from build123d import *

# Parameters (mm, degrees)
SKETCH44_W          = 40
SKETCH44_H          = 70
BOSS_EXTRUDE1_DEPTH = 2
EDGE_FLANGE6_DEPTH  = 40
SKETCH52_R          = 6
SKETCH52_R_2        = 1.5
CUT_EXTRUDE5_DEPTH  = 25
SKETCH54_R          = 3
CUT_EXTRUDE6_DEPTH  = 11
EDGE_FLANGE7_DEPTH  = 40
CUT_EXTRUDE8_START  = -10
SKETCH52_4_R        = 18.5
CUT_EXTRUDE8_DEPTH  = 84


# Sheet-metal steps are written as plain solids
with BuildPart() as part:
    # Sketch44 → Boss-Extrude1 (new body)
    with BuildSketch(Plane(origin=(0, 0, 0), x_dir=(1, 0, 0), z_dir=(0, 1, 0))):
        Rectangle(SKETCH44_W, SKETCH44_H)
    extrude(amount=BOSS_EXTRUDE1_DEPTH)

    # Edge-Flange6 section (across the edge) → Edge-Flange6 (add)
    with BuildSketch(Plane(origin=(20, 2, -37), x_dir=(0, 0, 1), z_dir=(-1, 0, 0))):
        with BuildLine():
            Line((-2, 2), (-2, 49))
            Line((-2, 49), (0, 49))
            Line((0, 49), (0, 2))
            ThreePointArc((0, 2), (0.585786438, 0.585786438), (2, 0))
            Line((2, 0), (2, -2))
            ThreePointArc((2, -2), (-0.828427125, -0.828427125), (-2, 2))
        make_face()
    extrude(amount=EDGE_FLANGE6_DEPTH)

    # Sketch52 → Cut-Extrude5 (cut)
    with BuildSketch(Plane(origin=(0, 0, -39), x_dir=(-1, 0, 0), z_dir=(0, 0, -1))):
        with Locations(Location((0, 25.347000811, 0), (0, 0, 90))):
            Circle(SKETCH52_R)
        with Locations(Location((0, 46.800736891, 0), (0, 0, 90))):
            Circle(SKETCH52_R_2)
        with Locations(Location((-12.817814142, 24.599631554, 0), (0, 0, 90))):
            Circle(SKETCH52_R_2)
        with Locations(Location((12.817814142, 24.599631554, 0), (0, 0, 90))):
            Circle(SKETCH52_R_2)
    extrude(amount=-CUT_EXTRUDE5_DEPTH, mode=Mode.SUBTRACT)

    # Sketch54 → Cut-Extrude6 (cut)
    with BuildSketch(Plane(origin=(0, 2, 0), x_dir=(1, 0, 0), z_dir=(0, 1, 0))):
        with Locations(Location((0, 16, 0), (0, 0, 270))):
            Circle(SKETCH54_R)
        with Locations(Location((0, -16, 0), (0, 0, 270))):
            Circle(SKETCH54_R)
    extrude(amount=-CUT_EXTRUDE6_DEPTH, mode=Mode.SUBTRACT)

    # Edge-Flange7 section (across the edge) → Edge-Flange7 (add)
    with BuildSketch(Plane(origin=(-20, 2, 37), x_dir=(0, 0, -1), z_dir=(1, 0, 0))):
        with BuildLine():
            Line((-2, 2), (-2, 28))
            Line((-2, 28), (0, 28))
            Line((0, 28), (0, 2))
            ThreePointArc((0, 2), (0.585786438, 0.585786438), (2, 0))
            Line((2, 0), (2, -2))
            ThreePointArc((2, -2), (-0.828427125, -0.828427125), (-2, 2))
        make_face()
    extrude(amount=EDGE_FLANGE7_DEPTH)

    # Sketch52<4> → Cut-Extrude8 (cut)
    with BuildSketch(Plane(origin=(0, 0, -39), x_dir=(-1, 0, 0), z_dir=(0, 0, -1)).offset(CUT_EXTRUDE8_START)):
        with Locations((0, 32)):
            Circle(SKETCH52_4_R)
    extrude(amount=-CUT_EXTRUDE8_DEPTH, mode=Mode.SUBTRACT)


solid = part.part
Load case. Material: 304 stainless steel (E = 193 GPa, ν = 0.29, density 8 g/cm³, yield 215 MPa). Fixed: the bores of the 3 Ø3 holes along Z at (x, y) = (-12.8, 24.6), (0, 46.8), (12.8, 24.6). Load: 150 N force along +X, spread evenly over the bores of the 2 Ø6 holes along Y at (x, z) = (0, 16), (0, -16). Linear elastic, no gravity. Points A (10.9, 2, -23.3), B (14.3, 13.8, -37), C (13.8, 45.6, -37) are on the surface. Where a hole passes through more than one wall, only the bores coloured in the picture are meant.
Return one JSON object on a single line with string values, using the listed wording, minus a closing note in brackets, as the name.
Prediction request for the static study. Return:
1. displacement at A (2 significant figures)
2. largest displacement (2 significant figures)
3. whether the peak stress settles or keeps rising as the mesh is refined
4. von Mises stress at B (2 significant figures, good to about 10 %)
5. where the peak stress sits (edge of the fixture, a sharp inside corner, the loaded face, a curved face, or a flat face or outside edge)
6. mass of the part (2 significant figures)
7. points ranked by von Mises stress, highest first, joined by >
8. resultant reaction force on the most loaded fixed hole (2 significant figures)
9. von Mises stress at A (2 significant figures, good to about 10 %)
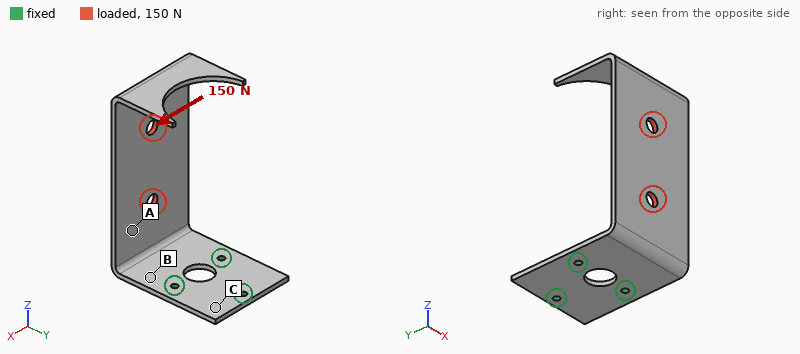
{"displacement at A": "0.15 mm", "largest displacement": "0.75 mm", "whether the peak stress settles or keeps rising as the mesh is refined": "keeps rising", "von Mises stress at B": "100 MPa", "where the peak stress sits": "edge of the fixture", "mass of the part": "87 g", "points ranked by von Mises stress, highest first, joined by >": "B > A > C", "resultant reaction force on the most loaded fixed hole": "240 N", "von Mises stress at A": "31 MPa"}
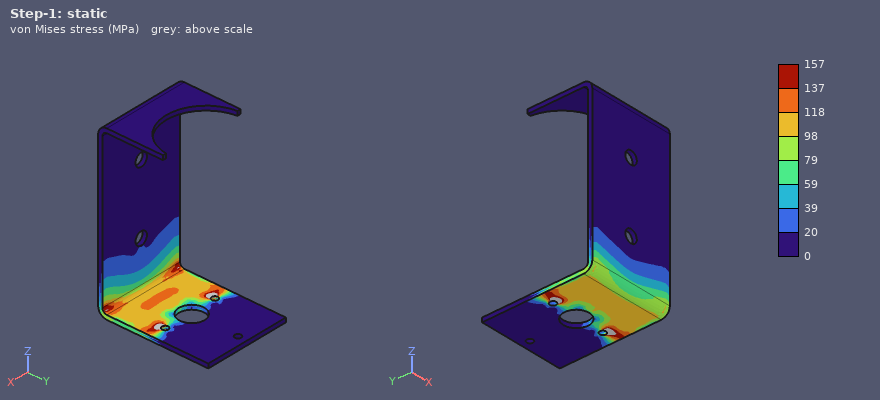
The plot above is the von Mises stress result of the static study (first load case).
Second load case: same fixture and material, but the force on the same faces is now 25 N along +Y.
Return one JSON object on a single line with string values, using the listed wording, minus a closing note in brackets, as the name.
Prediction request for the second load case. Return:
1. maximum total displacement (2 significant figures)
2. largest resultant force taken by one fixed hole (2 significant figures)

{"maximum total displacement": "0.61 mm", "largest resultant force taken by one fixed hole": "14 N"}
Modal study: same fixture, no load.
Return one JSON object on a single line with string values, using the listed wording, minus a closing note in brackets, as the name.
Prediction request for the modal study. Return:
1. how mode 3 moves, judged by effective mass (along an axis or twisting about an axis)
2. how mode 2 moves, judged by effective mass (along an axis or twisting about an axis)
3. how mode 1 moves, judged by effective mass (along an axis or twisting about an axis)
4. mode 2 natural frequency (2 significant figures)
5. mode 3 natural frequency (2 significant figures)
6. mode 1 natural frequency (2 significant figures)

{"how mode 3 moves, judged by effective mass": "along Z", "how mode 2 moves, judged by effective mass": "along X", "how mode 1 moves, judged by effective mass": "along Y", "mode 2 natural frequency": "320 Hz", "mode 3 natural frequency": "700 Hz", "mode 1 natural frequency": "140 Hz"}
